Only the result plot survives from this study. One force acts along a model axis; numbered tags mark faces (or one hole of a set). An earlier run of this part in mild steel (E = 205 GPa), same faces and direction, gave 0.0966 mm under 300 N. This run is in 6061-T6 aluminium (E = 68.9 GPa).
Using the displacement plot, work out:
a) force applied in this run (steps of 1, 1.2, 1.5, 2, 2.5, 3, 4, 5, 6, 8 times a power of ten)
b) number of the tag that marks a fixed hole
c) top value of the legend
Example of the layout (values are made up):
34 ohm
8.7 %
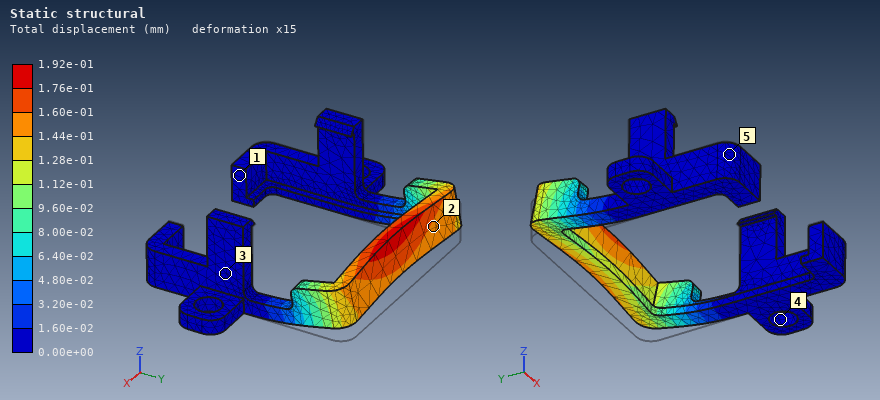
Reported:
200 N
4
1.92e-01 mm
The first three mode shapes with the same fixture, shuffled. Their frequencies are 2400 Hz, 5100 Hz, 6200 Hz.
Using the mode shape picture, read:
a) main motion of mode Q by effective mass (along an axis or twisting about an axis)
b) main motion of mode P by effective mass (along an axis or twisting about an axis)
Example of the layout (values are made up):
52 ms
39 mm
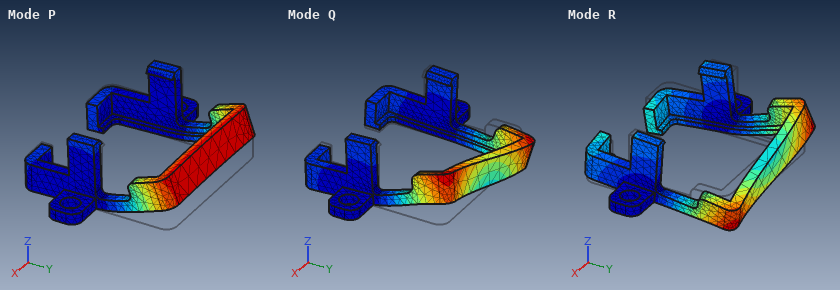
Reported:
along X
along Z
